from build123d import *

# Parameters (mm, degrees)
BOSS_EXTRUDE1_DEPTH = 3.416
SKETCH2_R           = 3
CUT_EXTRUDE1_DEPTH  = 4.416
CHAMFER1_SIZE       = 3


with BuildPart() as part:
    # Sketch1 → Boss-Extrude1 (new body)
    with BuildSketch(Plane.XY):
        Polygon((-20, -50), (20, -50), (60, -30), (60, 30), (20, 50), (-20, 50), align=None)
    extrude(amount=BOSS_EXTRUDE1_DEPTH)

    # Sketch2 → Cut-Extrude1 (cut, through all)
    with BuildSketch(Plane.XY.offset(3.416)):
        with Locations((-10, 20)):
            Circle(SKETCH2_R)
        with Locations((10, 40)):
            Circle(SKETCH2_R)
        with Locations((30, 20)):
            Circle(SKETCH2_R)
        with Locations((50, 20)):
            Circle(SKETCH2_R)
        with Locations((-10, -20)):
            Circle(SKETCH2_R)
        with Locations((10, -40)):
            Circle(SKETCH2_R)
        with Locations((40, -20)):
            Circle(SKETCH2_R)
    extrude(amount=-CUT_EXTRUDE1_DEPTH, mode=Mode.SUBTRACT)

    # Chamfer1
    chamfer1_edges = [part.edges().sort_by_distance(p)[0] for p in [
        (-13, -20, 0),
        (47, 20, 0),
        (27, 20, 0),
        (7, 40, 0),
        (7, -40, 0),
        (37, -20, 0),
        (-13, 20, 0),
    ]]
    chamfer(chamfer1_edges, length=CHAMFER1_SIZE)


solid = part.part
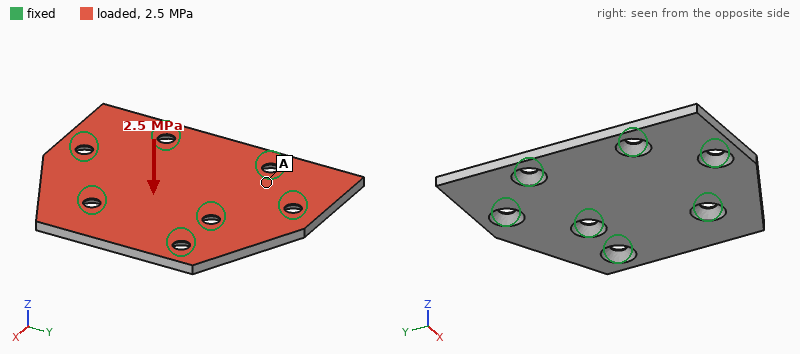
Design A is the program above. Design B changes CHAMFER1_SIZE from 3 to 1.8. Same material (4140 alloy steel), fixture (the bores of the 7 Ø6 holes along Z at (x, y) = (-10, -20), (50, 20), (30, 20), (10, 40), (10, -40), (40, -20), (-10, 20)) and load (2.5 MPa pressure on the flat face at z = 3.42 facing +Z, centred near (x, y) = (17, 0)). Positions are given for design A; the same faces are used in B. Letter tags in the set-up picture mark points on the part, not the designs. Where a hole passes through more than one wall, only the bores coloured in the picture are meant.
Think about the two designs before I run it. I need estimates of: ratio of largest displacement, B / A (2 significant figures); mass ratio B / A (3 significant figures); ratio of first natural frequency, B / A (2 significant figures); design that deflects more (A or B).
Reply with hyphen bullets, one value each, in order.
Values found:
- 0.83
- 1.02
- 1.2
- A
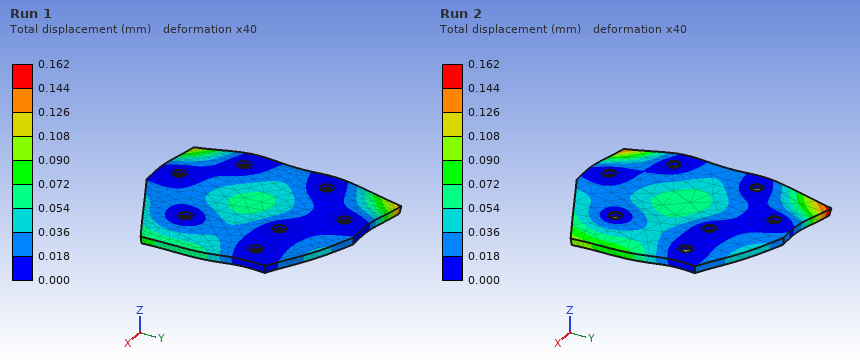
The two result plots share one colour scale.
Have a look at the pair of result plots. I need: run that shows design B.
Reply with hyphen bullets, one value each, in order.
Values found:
- Run 1
